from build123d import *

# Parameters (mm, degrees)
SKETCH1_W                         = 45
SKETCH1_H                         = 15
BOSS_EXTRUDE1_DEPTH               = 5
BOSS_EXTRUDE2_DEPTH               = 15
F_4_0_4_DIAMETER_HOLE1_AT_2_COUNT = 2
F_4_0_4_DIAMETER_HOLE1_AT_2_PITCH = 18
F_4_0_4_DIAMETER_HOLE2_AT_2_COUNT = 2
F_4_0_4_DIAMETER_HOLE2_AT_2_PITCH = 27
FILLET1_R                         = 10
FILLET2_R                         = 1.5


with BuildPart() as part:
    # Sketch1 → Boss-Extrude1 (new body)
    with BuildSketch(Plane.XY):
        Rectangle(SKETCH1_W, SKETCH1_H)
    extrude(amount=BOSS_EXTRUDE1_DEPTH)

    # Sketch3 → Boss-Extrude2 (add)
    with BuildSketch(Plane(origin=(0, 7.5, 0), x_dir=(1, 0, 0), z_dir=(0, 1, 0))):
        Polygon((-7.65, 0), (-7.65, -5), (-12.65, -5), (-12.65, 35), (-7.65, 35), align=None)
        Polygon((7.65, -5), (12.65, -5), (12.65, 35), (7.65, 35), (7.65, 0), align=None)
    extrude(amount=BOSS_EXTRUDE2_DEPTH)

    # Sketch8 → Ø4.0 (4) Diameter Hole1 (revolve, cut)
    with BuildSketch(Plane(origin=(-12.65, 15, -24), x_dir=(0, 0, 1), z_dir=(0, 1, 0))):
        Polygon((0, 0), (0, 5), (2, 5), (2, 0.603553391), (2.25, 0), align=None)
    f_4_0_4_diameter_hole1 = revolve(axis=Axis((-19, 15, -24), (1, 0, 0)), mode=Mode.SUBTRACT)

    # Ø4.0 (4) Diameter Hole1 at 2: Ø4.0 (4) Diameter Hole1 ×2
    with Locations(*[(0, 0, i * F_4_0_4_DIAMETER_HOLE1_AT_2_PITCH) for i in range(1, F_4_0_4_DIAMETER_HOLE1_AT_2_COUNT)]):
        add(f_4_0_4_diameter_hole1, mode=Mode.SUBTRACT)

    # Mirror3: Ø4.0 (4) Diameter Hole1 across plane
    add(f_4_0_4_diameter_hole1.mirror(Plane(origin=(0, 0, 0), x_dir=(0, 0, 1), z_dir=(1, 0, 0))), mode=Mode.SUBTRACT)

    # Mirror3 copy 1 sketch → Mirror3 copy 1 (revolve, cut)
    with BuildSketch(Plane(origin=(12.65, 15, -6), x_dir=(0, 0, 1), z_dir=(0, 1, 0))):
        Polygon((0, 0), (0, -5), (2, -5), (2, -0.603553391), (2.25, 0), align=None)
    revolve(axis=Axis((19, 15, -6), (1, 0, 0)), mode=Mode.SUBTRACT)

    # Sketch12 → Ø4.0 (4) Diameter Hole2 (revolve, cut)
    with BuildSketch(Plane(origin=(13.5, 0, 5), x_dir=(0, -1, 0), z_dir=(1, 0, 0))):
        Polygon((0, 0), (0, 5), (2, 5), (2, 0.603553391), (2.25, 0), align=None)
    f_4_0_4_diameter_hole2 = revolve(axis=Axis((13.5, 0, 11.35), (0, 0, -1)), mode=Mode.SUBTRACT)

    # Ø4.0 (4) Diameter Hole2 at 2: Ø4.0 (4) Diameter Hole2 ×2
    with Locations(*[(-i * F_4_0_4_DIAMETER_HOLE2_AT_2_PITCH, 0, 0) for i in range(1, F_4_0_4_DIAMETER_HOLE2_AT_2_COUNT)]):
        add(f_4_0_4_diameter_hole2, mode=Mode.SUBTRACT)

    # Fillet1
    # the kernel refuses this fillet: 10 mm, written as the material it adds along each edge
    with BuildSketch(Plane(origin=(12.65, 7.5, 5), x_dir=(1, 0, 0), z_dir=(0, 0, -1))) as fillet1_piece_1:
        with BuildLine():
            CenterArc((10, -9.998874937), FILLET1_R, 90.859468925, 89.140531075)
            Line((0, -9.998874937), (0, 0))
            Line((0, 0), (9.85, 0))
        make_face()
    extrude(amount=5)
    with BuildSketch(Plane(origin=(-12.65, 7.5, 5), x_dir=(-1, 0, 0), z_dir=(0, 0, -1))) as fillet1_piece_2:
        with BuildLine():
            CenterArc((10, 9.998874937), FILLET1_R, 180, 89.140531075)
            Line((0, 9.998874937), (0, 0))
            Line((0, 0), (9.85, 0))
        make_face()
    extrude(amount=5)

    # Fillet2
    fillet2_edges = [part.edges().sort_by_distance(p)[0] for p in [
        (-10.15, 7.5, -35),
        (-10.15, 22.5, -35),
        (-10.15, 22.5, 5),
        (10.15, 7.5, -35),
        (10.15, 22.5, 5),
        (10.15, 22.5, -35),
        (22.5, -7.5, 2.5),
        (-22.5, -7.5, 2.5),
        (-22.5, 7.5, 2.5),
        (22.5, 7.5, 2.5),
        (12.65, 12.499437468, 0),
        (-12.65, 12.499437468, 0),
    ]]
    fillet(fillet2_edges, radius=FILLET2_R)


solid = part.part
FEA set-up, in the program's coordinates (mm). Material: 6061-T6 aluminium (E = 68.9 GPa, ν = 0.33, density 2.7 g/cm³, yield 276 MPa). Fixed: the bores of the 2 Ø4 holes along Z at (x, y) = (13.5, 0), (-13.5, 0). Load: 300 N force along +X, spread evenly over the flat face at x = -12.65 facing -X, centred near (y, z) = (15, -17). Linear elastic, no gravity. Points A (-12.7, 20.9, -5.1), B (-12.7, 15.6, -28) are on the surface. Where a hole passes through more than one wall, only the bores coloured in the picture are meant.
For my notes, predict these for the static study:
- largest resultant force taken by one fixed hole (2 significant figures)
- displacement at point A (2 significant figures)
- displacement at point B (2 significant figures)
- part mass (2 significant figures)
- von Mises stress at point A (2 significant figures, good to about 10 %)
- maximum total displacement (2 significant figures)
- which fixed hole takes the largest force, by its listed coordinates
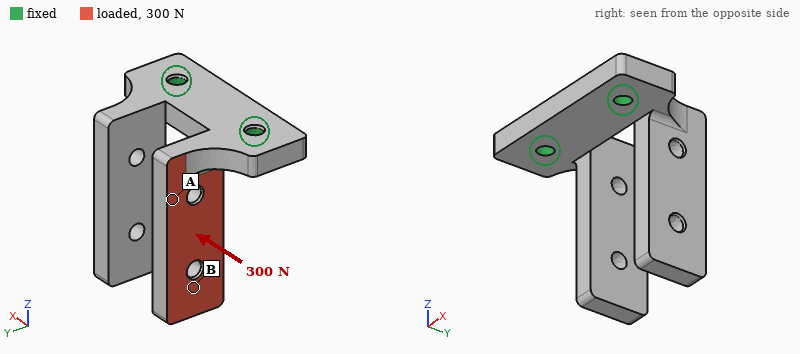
290 N
0.072 mm
0.32 mm
25 g
57 MPa
0.43 mm
(-13.5, 0)
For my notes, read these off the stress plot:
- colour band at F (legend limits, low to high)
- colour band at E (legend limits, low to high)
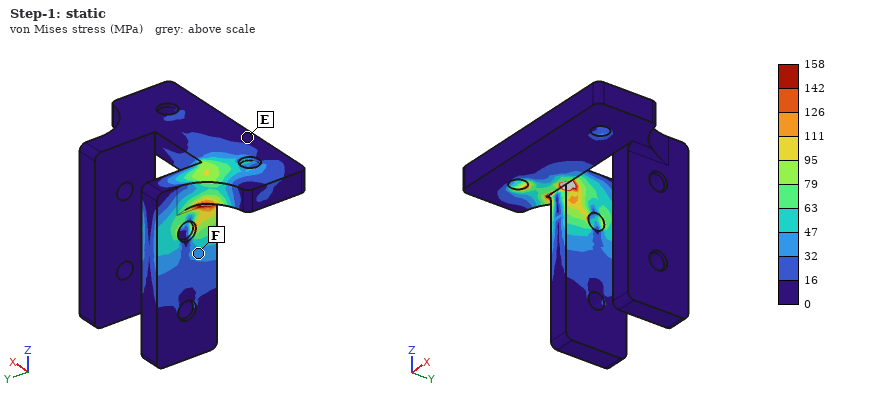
32 to 47 MPa
0 to 16 MPa
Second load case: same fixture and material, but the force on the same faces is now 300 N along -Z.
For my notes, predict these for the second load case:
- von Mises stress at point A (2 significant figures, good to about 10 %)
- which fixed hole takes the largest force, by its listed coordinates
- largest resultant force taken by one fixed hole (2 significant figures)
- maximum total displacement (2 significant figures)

13 MPa
(-13.5, 0)
310 N
0.16 mm
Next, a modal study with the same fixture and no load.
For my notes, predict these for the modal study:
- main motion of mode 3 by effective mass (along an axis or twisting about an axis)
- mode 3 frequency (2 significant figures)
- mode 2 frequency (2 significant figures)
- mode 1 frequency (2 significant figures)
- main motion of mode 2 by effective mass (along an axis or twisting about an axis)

along Y
2100 Hz
2000 Hz
1900 Hz
along X
